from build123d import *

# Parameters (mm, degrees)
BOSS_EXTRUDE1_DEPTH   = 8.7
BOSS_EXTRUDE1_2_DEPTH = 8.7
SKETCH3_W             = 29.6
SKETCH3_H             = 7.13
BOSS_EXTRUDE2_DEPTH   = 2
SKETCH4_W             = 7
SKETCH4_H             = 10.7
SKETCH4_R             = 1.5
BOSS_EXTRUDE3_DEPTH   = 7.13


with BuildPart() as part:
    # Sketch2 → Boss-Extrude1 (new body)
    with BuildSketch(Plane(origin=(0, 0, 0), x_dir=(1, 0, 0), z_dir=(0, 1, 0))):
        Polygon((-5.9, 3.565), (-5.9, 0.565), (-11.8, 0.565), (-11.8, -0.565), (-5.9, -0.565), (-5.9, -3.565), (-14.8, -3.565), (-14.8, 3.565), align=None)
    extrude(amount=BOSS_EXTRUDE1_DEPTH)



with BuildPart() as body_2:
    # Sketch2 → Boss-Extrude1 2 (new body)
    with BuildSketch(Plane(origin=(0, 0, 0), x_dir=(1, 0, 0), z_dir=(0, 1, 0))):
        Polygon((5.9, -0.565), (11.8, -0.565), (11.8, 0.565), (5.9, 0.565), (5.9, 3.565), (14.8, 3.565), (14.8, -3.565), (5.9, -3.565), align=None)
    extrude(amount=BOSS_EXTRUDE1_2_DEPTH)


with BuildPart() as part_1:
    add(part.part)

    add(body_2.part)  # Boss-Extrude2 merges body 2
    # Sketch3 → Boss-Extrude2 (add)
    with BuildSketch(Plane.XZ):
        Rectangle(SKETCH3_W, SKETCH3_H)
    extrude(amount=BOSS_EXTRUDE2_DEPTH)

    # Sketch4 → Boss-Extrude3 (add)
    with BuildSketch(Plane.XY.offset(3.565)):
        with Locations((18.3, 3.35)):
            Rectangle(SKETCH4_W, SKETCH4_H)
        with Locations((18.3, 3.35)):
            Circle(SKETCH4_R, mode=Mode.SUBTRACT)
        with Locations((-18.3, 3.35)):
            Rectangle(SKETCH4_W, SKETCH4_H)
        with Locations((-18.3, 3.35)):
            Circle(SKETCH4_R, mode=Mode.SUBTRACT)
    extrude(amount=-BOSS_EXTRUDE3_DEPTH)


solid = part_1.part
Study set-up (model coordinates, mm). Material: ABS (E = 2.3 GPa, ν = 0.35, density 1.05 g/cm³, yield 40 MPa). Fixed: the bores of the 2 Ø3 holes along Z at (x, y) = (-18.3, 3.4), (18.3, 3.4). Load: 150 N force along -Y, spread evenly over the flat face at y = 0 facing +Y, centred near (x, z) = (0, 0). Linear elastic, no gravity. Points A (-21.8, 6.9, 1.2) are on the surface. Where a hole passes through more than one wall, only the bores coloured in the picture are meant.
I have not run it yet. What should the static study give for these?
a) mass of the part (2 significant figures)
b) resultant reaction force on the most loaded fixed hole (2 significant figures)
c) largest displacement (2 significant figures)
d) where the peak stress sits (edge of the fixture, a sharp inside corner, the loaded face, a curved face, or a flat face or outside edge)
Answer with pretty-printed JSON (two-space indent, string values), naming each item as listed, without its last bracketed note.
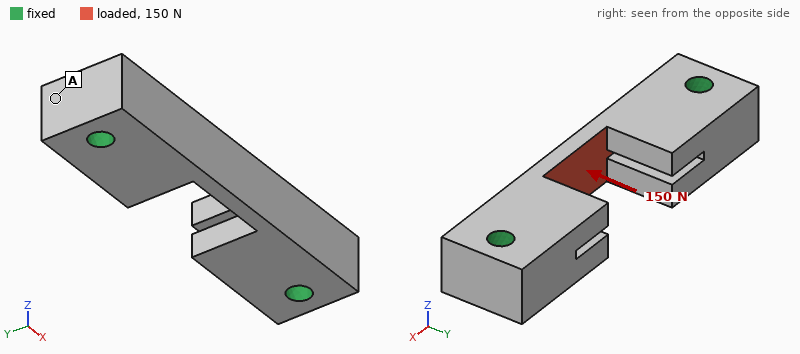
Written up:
{
  "mass of the part": "2.5 g",
  "resultant reaction force on the most loaded fixed hole": "110 N",
  "largest displacement": "0.20 mm",
  "where the peak stress sits": "a flat face or outside edge"
}
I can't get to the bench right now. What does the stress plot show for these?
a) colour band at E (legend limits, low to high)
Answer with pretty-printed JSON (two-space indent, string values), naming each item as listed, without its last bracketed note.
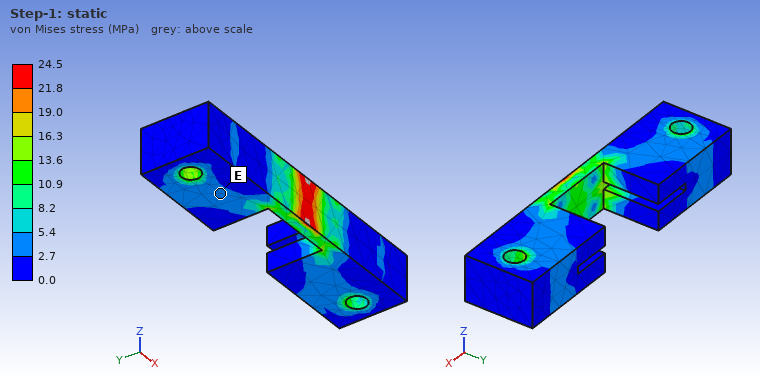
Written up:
{
  "colour band at E": "2.7 to 5.4 MPa"
}
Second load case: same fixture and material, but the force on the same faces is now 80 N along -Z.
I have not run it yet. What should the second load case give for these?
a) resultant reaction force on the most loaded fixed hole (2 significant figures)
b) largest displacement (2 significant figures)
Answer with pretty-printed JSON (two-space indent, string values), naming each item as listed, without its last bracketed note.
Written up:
{
  "resultant reaction force on the most loaded fixed hole": "40 N",
  "largest displacement": "95 µm"
}
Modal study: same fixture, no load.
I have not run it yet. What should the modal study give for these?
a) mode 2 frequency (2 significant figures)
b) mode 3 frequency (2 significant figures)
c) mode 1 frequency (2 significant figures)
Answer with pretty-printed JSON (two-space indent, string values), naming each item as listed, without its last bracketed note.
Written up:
{
  "mode 2 frequency": "7800 Hz",
  "mode 3 frequency": "8200 Hz",
  "mode 1 frequency": "7800 Hz"
}
